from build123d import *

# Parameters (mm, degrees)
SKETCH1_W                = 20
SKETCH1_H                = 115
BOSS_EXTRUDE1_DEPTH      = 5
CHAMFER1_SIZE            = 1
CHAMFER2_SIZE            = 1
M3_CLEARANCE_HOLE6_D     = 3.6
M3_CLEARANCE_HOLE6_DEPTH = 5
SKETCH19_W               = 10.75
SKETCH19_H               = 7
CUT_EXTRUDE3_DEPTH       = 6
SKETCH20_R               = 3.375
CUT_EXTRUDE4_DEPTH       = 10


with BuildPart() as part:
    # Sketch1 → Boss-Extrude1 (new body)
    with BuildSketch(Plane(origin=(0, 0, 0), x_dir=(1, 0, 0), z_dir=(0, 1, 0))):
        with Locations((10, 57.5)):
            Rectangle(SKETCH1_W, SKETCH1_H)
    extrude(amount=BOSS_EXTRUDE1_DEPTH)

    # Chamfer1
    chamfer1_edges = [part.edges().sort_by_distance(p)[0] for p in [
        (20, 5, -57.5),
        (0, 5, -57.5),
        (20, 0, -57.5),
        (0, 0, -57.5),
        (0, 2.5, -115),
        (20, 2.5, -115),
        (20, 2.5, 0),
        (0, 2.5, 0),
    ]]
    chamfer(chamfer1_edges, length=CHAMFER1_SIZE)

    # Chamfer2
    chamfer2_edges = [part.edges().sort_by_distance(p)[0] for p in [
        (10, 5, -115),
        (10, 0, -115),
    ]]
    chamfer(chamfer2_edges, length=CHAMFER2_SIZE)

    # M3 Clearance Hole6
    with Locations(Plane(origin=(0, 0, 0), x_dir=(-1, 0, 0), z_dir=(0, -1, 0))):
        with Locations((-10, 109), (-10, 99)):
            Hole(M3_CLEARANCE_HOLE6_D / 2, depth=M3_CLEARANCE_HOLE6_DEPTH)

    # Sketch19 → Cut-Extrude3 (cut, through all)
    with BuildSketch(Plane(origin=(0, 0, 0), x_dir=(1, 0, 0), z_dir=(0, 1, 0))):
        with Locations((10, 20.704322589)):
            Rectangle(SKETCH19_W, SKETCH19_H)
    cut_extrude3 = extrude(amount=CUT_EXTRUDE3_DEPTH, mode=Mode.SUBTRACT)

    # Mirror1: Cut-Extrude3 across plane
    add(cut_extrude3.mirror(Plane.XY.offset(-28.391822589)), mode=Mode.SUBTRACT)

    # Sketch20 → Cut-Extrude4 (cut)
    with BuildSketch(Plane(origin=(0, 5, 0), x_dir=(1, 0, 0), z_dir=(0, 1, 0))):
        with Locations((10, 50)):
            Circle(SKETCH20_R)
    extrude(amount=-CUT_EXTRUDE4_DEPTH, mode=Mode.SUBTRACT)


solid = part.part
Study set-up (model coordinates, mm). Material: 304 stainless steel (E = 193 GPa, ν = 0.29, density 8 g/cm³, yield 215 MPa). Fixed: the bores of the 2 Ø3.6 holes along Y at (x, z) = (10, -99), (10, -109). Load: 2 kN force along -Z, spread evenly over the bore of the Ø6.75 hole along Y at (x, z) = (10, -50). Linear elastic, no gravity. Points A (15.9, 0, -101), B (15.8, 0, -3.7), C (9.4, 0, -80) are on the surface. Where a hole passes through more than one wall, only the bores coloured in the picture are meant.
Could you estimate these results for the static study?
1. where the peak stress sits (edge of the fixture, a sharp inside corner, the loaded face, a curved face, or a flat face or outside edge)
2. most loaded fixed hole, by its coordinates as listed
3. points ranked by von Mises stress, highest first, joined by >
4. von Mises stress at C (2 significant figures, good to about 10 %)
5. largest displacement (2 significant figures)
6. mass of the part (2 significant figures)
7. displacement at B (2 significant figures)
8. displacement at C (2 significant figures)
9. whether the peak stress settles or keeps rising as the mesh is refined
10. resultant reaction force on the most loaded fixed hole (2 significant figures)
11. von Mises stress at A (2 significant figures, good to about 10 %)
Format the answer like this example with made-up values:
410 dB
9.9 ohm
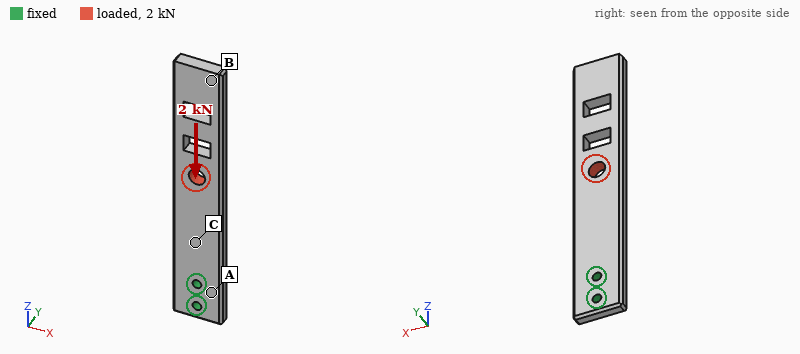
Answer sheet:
edge of the fixture
(10, -99)
C > A > B
21 MPa
6.6 µm
82 g
5.7 µm
2.4 µm
keeps rising
1.6 kN
12 MPa
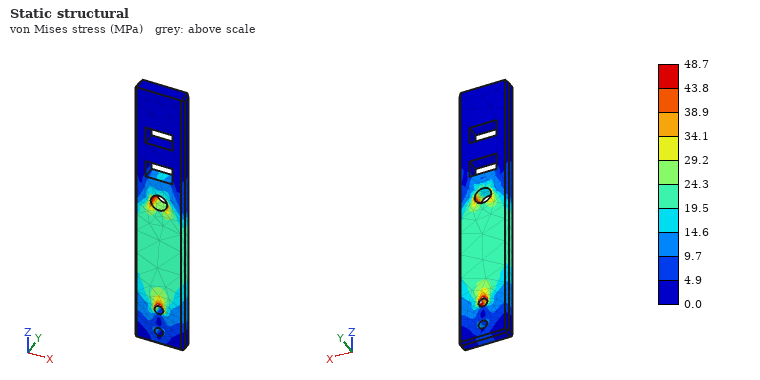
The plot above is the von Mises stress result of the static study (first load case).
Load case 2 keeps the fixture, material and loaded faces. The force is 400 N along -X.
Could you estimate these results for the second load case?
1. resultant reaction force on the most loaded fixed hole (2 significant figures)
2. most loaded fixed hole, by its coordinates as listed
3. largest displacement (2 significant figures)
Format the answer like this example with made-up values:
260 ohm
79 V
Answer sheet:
1.7 kN
(10, -99)
0.10 mm
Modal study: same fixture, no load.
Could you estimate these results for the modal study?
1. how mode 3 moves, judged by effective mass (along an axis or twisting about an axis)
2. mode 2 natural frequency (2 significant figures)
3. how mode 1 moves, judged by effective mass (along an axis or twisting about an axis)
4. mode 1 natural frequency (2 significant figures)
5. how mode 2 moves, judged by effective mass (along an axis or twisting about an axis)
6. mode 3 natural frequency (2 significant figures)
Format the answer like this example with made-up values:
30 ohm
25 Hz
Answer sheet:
along Y
1400 Hz
along Y
420 Hz
along X
2200 Hz
